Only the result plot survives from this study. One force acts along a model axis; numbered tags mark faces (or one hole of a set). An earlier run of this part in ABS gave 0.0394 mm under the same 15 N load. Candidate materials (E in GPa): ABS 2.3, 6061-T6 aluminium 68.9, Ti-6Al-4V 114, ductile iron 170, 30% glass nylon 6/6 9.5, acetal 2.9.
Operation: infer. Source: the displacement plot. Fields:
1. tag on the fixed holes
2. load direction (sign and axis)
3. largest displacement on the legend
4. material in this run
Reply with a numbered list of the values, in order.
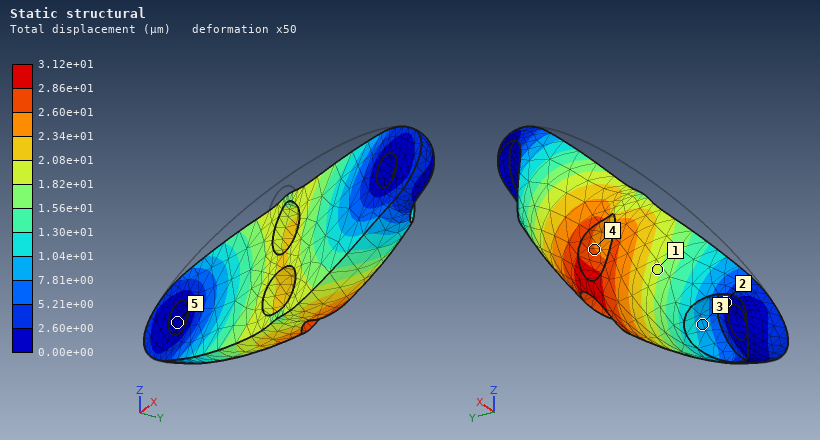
1. 5
2. -Z
3. 3.12e+01 µm
4. acetal
